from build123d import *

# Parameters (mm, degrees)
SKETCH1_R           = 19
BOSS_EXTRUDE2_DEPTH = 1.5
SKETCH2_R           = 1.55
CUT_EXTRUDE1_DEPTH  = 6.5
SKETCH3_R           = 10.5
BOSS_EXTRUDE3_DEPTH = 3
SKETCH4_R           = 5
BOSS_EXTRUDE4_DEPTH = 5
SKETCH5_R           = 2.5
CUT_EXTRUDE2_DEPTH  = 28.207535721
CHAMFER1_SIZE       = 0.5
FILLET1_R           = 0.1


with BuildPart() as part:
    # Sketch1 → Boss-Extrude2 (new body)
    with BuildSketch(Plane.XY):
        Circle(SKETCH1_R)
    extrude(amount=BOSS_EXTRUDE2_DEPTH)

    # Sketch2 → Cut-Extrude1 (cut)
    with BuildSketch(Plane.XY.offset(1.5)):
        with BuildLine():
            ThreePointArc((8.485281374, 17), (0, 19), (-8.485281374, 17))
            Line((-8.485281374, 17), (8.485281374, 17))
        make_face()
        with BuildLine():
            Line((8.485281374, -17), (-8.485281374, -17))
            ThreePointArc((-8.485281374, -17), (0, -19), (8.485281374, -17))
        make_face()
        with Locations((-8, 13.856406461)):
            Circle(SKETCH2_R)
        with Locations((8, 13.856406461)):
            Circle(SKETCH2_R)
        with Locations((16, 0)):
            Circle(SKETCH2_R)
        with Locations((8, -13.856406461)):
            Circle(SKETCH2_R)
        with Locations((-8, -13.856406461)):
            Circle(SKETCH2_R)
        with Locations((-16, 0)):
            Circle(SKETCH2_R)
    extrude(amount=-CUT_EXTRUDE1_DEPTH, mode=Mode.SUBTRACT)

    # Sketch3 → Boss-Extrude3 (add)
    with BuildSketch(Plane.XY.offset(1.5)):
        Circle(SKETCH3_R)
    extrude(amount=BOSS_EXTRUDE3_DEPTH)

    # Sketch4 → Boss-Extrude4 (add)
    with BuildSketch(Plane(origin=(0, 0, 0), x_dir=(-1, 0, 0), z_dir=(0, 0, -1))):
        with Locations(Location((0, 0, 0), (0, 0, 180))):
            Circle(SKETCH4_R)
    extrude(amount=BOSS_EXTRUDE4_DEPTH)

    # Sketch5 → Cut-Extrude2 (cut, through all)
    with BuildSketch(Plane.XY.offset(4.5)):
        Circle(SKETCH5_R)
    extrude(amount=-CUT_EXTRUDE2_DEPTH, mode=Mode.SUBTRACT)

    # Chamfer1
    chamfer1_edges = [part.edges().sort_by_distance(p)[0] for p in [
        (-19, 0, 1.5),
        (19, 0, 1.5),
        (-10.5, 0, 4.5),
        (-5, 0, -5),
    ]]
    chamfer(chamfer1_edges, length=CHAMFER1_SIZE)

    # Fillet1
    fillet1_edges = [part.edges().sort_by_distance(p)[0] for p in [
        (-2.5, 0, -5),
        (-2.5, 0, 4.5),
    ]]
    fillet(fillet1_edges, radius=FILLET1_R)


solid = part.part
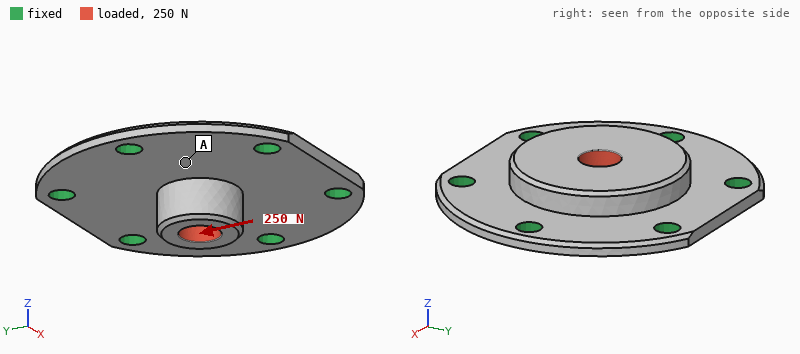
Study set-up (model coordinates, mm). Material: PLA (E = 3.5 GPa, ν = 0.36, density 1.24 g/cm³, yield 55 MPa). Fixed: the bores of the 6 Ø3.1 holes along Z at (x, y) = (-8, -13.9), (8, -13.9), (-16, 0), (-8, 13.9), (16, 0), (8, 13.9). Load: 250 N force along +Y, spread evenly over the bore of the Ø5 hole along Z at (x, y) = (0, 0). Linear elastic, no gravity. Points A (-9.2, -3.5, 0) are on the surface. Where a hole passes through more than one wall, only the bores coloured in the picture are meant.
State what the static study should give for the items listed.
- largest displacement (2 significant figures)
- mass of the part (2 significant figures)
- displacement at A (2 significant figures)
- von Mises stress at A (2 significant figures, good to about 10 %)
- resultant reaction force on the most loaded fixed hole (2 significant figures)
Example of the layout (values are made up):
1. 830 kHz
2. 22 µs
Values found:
1. 42 µm
2. 3.5 g
3. 9.4 µm
4. 3.1 MPa
5. 54 N
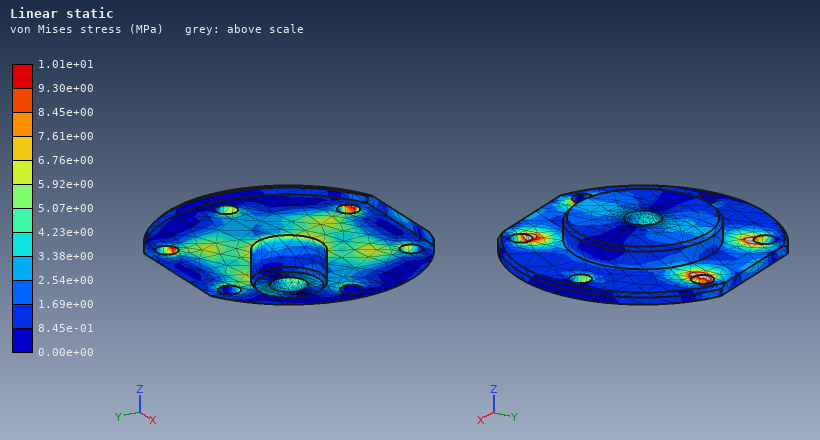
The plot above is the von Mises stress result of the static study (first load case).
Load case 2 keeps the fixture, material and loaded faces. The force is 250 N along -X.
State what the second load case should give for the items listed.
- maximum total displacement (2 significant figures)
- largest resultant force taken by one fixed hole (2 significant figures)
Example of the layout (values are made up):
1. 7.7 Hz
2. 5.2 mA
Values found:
1. 41 µm
2. 60 N
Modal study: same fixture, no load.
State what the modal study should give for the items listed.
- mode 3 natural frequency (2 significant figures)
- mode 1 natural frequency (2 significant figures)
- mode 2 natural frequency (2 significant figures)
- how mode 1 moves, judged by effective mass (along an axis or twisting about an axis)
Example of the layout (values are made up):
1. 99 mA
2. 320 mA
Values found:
1. 9000 Hz
2. 5500 Hz
3. 9000 Hz
4. along Z
